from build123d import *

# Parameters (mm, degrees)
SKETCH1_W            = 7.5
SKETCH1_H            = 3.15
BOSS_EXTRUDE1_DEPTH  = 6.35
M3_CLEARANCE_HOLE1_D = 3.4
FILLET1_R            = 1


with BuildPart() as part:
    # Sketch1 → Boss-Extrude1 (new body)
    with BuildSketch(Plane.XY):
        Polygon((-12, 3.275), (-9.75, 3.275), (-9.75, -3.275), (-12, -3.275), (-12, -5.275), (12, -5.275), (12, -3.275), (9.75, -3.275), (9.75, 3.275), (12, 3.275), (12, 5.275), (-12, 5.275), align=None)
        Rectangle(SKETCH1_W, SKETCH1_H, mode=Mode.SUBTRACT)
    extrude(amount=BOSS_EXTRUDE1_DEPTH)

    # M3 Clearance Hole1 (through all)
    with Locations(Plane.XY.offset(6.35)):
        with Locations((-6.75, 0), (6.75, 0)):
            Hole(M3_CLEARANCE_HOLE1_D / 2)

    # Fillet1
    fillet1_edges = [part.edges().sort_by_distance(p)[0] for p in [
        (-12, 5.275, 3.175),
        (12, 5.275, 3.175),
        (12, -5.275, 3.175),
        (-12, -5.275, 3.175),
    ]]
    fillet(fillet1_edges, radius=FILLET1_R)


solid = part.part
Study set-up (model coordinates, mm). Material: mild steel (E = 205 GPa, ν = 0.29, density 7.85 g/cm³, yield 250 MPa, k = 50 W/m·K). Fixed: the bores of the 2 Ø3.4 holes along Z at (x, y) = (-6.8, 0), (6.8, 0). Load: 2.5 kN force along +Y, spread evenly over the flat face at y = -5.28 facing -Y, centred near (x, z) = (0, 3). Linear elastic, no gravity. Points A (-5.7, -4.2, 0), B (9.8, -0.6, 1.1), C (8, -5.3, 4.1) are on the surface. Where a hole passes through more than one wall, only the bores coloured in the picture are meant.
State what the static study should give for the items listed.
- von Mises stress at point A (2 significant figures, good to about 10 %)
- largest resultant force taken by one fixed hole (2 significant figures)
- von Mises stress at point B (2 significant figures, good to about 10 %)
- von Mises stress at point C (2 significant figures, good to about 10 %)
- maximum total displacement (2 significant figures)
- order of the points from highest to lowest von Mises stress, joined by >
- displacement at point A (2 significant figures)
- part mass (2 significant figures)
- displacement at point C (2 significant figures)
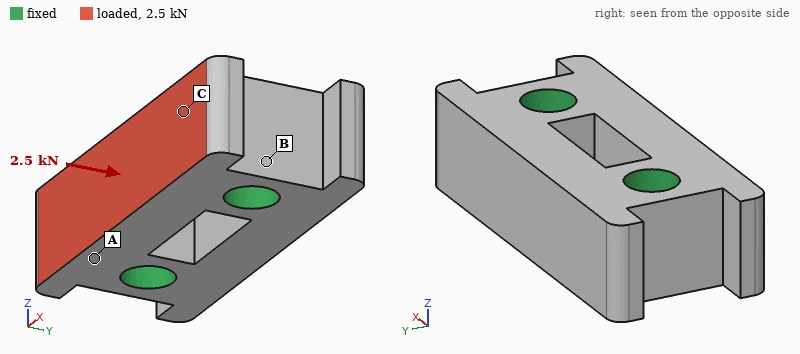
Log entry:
25 MPa
1.3 kN
12 MPa
37 MPa
1.8 µm
C > A > B
0.38 µm
9.0 g
0.46 µm
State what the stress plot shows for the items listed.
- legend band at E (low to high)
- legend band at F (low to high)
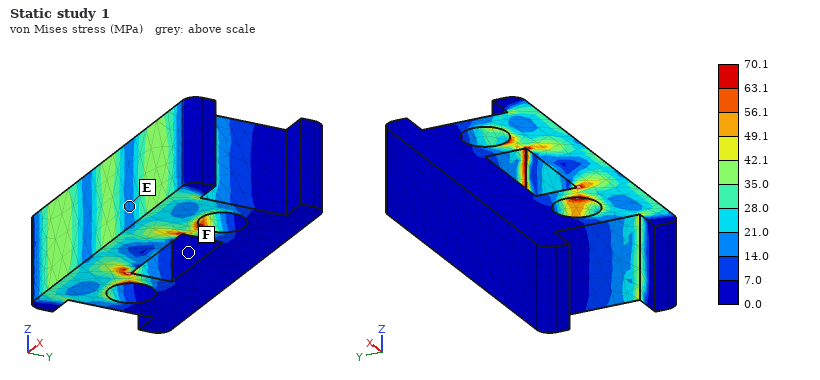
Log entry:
14.0 to 21.0 MPa
0.0 to 7.0 MPa
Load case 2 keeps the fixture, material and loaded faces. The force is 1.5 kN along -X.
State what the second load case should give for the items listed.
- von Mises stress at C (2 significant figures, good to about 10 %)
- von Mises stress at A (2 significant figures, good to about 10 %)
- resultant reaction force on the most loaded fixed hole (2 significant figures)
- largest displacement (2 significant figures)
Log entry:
32 MPa
22 MPa
800 N
2.5 µm
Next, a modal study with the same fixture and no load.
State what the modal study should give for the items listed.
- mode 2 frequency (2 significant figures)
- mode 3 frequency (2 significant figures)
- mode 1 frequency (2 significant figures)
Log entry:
92 kHz
94 kHz
91 kHz
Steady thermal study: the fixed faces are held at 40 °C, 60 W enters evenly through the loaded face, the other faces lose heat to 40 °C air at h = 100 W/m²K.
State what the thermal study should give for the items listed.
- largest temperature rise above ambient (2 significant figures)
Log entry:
69 K
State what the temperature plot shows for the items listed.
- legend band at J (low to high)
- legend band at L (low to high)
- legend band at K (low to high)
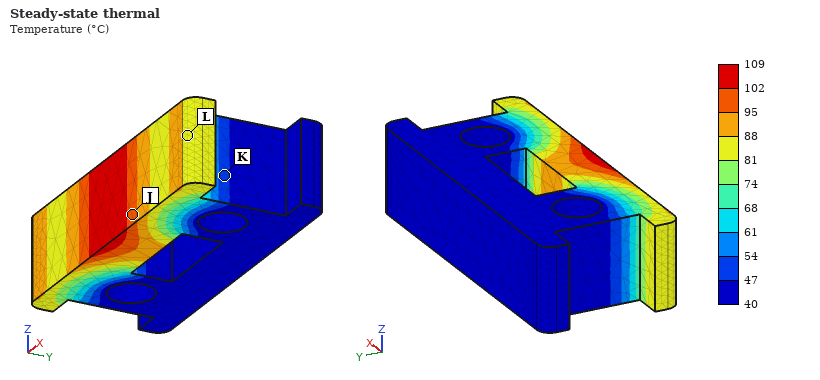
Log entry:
95 to 102 °C
81 to 88 °C
47 to 54 °C
